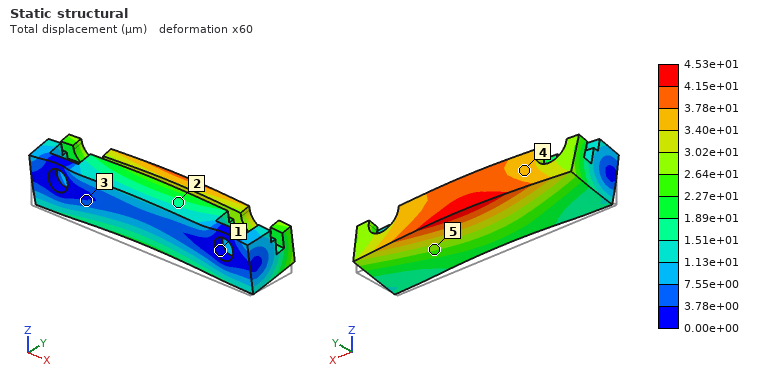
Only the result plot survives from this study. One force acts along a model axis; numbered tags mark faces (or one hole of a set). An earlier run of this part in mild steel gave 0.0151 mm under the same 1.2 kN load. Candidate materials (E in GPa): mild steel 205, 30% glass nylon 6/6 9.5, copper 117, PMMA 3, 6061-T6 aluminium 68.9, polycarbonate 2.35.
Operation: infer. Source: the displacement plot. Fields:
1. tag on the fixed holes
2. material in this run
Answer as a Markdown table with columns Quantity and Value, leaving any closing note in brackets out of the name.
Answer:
| Quantity | Value |
|---|---|
| tag on the fixed holes | 1 |
| material in this run | 6061-T6 aluminium |
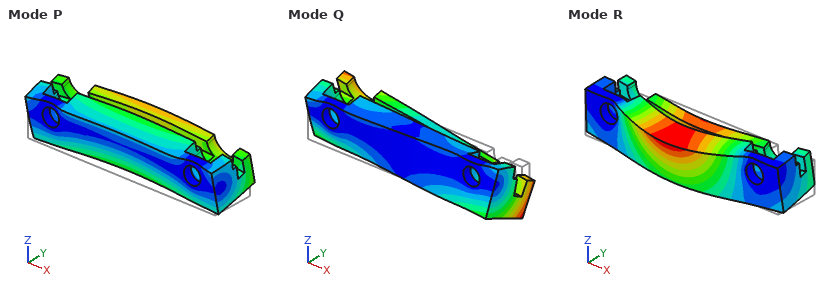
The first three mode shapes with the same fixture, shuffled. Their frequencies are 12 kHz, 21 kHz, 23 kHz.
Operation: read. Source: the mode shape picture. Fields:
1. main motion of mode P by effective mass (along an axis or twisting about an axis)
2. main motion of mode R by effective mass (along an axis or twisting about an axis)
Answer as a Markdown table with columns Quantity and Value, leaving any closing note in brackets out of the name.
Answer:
| Quantity | Value |
|---|---|
| main motion of mode P by effective mass | along Z |
| main motion of mode R by effective mass | along Y |
